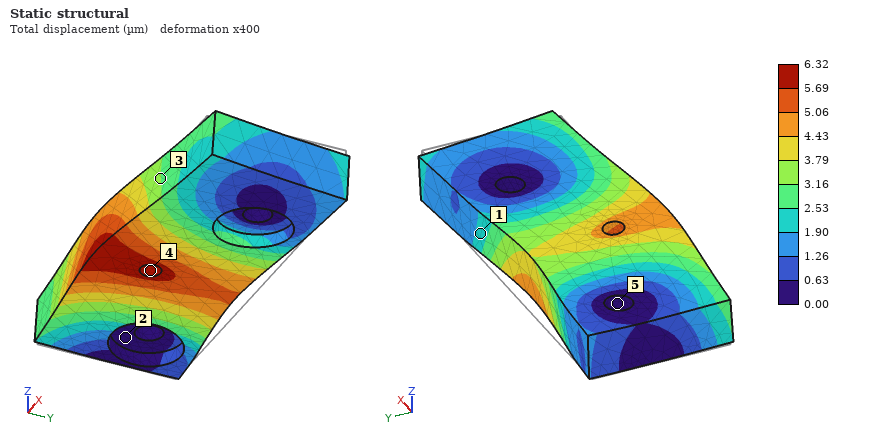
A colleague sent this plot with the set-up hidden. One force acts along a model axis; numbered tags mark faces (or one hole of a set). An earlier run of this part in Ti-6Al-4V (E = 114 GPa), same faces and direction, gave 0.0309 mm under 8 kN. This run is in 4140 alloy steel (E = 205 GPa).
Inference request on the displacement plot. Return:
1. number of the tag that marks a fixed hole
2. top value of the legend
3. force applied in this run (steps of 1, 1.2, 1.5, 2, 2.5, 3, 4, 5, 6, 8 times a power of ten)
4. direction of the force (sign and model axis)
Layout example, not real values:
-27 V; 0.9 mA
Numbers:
5; 6.32 µm; 3 kN; -Y
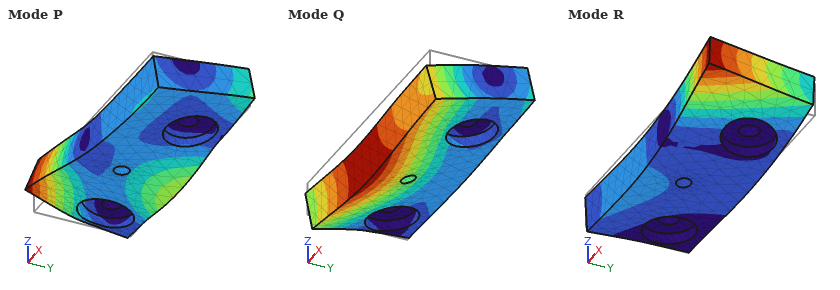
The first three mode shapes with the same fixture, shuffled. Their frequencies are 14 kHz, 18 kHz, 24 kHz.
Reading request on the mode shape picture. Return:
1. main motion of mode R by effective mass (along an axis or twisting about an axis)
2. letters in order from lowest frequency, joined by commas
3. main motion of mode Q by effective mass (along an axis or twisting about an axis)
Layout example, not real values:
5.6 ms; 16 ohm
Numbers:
twisting about Y; Q, R, P; along Z
